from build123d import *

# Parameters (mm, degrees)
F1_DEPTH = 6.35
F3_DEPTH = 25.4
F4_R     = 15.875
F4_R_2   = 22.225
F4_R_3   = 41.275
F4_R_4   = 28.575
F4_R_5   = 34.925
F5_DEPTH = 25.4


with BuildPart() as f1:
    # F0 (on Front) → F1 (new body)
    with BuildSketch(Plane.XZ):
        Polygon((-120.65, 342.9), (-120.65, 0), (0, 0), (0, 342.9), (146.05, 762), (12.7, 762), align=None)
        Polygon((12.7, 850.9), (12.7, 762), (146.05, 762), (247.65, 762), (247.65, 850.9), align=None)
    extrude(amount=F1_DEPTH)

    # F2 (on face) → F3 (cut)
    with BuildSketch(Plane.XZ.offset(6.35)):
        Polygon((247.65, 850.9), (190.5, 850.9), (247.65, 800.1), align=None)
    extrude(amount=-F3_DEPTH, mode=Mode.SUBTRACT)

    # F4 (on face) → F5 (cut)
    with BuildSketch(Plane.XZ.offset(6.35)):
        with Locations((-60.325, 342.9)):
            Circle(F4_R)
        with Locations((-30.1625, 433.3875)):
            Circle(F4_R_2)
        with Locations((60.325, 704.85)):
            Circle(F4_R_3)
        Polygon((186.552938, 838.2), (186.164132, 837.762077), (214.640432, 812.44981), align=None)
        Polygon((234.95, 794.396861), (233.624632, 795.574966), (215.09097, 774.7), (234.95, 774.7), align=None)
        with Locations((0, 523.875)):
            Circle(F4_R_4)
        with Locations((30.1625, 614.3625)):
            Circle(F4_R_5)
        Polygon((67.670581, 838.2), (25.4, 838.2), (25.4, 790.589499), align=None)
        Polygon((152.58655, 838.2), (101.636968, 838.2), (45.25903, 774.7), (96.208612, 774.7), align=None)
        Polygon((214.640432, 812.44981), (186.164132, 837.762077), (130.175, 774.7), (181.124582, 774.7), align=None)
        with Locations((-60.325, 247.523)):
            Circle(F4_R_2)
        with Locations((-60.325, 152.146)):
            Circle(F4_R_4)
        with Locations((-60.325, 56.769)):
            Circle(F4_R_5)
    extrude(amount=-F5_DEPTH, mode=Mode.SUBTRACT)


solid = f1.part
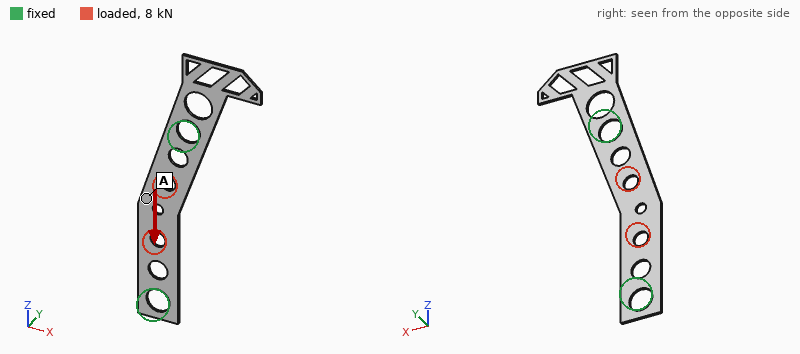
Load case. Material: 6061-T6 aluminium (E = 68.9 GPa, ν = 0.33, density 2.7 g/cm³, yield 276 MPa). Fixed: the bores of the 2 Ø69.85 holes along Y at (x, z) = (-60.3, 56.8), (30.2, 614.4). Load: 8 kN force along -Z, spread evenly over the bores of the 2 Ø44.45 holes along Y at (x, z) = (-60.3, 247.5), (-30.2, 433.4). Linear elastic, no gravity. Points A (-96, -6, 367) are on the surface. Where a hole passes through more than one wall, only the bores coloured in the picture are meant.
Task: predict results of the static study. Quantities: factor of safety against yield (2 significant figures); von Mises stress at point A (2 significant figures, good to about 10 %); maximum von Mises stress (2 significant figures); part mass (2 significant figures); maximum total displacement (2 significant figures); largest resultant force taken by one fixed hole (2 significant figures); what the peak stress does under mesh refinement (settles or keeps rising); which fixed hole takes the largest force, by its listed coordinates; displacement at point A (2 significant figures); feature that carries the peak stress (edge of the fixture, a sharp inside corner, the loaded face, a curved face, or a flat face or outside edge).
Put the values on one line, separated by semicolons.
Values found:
10; 2.3 MPa; 27 MPa; 1.5 kg; 38 µm; 4.5 kN; settles; (-60.3, 56.8); 34 µm; a curved face
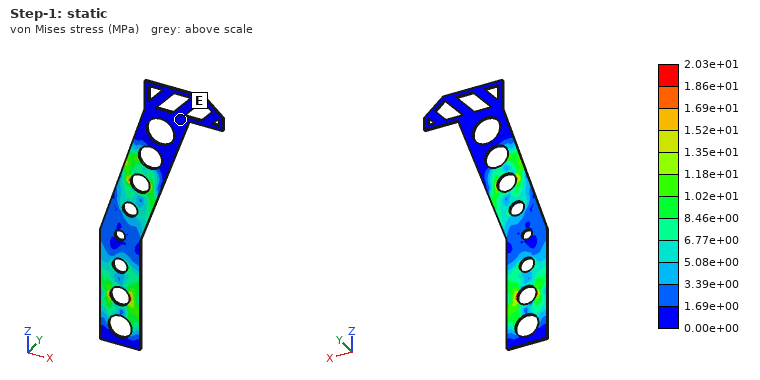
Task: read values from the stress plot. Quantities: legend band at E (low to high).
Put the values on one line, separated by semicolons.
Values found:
0.00e+00 to 1.69e+00 MPa
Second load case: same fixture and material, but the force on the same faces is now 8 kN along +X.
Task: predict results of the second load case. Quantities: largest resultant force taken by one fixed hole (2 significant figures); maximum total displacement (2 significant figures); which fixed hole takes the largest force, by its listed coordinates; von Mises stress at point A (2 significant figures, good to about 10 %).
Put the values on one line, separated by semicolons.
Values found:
5.3 kN; 0.16 mm; (30.2, 614.4); 14 MPa
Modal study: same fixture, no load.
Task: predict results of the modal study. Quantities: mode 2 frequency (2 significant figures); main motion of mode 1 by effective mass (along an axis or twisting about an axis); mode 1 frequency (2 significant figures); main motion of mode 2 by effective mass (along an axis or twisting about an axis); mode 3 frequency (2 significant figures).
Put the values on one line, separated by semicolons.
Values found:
120 Hz; along Y; 69 Hz; along Y; 180 Hz
